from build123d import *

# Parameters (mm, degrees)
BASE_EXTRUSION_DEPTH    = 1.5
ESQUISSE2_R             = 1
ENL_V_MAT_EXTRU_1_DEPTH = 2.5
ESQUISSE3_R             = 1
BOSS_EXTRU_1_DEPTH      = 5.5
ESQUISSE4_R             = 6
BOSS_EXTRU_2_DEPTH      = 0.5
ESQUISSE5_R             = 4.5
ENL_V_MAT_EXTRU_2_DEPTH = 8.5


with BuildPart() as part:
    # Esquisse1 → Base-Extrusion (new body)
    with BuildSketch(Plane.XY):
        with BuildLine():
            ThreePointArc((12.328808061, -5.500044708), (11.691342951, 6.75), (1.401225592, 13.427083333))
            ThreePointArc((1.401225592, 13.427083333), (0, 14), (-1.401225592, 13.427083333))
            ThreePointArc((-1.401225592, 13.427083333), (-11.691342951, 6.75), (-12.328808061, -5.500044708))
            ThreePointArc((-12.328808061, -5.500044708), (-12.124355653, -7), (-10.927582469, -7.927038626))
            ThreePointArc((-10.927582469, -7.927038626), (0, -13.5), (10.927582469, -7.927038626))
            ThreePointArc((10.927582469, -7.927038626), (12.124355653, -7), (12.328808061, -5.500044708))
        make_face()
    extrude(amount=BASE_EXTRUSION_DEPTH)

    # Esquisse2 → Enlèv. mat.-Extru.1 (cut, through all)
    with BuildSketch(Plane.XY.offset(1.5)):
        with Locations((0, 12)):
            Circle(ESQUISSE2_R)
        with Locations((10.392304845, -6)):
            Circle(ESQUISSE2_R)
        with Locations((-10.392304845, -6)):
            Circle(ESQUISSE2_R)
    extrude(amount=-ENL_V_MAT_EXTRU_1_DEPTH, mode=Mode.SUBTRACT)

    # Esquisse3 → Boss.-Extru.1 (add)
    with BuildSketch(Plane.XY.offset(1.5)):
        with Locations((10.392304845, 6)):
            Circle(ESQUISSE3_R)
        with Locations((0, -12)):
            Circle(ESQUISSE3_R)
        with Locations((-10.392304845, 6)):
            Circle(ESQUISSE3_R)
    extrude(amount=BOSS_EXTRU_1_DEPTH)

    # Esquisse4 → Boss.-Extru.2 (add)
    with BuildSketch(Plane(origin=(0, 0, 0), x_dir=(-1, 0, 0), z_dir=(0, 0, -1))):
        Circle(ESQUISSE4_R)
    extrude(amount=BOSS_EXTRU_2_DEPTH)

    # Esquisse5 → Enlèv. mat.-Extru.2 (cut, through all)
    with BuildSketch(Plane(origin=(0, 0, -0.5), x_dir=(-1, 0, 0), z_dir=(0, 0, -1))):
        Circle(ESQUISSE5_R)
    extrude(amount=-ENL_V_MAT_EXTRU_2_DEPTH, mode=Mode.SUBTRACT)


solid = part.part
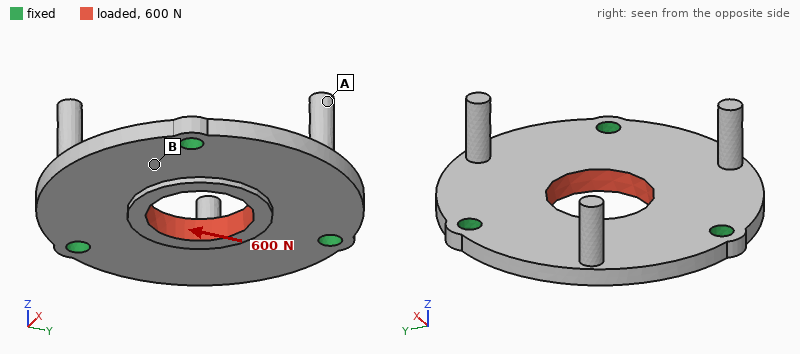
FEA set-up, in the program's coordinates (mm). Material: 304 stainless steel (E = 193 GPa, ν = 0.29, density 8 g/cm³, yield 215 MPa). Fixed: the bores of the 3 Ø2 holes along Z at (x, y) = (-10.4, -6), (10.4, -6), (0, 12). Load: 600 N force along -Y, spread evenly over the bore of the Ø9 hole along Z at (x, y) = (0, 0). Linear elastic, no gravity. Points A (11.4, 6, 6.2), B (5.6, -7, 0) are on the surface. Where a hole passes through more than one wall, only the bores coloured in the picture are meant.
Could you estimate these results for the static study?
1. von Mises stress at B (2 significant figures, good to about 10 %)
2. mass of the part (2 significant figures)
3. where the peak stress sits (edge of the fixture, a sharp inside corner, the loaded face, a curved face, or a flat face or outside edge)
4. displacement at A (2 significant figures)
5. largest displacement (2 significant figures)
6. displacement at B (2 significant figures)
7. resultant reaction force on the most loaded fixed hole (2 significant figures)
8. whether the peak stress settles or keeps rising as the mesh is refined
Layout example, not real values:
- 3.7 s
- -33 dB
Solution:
- 14 MPa
- 6.6 g
- edge of the fixture
- 0.67 µm
- 1.8 µm
- 0.99 µm
- 200 N
- keeps rising
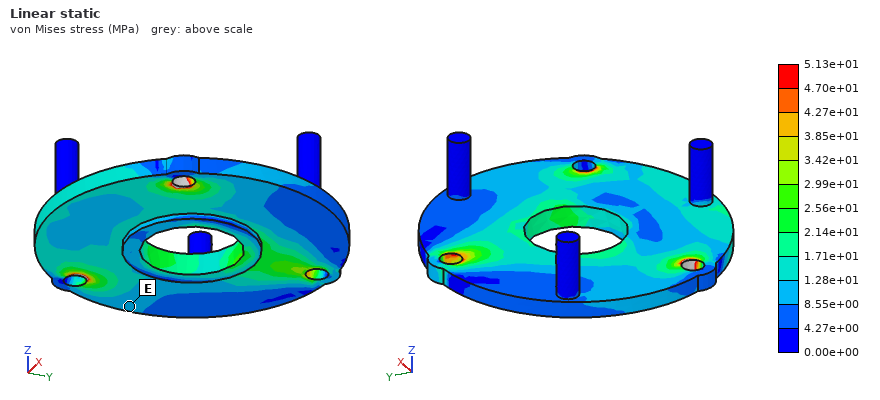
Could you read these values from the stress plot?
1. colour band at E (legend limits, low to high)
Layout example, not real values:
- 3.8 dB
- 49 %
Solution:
- 8.55e+00 to 1.28e+01 MPa
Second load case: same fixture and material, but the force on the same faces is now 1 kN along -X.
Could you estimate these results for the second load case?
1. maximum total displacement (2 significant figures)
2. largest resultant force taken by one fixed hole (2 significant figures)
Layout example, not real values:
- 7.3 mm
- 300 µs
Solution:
- 2.8 µm
- 340 N
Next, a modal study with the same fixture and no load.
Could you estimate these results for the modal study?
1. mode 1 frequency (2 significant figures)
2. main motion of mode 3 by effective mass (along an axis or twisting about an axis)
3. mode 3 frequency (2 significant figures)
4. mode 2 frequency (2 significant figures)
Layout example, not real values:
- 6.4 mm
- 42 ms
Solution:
- 12 kHz
- along Z
- 13 kHz
- 12 kHz
